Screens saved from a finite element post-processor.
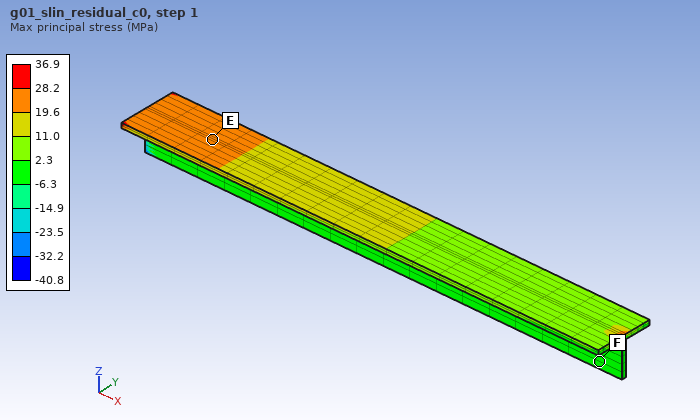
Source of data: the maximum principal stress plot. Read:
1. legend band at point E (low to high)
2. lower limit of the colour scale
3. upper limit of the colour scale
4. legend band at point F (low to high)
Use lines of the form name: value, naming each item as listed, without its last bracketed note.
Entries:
legend band at point E: 19.6 to 28.2 MPa
lower limit of the colour scale: -40.8 MPa
upper limit of the colour scale: 36.9 MPa
legend band at point F: -6.3 to 2.3 MPa
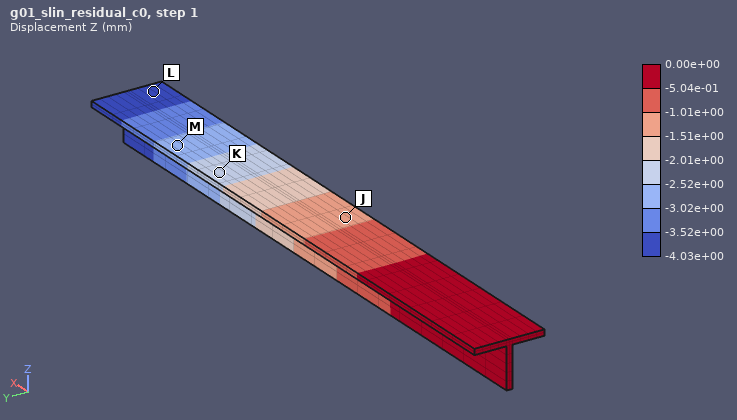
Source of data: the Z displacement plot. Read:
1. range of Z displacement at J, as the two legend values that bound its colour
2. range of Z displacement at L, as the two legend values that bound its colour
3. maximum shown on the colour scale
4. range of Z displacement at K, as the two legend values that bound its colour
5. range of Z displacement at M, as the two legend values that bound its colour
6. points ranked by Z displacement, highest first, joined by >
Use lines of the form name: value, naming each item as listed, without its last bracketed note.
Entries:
range of Z displacement at J, as the two legend values that bound its colour: -1.51e+00 to -1.01e+00 mm
range of Z displacement at L, as the two legend values that bound its colour: -4.03e+00 to -3.52e+00 mm
maximum shown on the colour scale: 0.00e+00 mm
range of Z displacement at K, as the two legend values that bound its colour: -2.52e+00 to -2.01e+00 mm
range of Z displacement at M, as the two legend values that bound its colour: -3.02e+00 to -2.52e+00 mm
points ranked by Z displacement, highest first, joined by >: J > K > M > L
